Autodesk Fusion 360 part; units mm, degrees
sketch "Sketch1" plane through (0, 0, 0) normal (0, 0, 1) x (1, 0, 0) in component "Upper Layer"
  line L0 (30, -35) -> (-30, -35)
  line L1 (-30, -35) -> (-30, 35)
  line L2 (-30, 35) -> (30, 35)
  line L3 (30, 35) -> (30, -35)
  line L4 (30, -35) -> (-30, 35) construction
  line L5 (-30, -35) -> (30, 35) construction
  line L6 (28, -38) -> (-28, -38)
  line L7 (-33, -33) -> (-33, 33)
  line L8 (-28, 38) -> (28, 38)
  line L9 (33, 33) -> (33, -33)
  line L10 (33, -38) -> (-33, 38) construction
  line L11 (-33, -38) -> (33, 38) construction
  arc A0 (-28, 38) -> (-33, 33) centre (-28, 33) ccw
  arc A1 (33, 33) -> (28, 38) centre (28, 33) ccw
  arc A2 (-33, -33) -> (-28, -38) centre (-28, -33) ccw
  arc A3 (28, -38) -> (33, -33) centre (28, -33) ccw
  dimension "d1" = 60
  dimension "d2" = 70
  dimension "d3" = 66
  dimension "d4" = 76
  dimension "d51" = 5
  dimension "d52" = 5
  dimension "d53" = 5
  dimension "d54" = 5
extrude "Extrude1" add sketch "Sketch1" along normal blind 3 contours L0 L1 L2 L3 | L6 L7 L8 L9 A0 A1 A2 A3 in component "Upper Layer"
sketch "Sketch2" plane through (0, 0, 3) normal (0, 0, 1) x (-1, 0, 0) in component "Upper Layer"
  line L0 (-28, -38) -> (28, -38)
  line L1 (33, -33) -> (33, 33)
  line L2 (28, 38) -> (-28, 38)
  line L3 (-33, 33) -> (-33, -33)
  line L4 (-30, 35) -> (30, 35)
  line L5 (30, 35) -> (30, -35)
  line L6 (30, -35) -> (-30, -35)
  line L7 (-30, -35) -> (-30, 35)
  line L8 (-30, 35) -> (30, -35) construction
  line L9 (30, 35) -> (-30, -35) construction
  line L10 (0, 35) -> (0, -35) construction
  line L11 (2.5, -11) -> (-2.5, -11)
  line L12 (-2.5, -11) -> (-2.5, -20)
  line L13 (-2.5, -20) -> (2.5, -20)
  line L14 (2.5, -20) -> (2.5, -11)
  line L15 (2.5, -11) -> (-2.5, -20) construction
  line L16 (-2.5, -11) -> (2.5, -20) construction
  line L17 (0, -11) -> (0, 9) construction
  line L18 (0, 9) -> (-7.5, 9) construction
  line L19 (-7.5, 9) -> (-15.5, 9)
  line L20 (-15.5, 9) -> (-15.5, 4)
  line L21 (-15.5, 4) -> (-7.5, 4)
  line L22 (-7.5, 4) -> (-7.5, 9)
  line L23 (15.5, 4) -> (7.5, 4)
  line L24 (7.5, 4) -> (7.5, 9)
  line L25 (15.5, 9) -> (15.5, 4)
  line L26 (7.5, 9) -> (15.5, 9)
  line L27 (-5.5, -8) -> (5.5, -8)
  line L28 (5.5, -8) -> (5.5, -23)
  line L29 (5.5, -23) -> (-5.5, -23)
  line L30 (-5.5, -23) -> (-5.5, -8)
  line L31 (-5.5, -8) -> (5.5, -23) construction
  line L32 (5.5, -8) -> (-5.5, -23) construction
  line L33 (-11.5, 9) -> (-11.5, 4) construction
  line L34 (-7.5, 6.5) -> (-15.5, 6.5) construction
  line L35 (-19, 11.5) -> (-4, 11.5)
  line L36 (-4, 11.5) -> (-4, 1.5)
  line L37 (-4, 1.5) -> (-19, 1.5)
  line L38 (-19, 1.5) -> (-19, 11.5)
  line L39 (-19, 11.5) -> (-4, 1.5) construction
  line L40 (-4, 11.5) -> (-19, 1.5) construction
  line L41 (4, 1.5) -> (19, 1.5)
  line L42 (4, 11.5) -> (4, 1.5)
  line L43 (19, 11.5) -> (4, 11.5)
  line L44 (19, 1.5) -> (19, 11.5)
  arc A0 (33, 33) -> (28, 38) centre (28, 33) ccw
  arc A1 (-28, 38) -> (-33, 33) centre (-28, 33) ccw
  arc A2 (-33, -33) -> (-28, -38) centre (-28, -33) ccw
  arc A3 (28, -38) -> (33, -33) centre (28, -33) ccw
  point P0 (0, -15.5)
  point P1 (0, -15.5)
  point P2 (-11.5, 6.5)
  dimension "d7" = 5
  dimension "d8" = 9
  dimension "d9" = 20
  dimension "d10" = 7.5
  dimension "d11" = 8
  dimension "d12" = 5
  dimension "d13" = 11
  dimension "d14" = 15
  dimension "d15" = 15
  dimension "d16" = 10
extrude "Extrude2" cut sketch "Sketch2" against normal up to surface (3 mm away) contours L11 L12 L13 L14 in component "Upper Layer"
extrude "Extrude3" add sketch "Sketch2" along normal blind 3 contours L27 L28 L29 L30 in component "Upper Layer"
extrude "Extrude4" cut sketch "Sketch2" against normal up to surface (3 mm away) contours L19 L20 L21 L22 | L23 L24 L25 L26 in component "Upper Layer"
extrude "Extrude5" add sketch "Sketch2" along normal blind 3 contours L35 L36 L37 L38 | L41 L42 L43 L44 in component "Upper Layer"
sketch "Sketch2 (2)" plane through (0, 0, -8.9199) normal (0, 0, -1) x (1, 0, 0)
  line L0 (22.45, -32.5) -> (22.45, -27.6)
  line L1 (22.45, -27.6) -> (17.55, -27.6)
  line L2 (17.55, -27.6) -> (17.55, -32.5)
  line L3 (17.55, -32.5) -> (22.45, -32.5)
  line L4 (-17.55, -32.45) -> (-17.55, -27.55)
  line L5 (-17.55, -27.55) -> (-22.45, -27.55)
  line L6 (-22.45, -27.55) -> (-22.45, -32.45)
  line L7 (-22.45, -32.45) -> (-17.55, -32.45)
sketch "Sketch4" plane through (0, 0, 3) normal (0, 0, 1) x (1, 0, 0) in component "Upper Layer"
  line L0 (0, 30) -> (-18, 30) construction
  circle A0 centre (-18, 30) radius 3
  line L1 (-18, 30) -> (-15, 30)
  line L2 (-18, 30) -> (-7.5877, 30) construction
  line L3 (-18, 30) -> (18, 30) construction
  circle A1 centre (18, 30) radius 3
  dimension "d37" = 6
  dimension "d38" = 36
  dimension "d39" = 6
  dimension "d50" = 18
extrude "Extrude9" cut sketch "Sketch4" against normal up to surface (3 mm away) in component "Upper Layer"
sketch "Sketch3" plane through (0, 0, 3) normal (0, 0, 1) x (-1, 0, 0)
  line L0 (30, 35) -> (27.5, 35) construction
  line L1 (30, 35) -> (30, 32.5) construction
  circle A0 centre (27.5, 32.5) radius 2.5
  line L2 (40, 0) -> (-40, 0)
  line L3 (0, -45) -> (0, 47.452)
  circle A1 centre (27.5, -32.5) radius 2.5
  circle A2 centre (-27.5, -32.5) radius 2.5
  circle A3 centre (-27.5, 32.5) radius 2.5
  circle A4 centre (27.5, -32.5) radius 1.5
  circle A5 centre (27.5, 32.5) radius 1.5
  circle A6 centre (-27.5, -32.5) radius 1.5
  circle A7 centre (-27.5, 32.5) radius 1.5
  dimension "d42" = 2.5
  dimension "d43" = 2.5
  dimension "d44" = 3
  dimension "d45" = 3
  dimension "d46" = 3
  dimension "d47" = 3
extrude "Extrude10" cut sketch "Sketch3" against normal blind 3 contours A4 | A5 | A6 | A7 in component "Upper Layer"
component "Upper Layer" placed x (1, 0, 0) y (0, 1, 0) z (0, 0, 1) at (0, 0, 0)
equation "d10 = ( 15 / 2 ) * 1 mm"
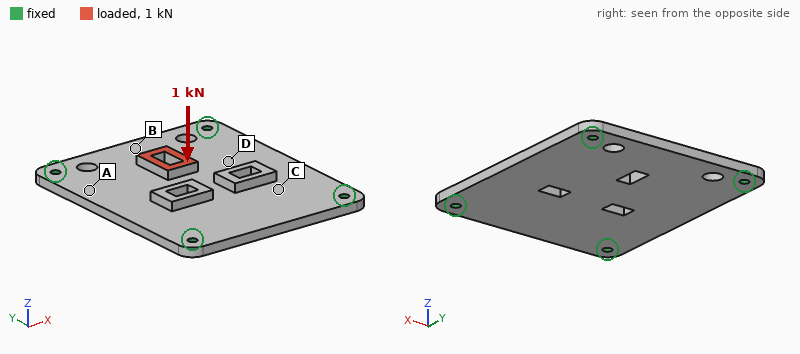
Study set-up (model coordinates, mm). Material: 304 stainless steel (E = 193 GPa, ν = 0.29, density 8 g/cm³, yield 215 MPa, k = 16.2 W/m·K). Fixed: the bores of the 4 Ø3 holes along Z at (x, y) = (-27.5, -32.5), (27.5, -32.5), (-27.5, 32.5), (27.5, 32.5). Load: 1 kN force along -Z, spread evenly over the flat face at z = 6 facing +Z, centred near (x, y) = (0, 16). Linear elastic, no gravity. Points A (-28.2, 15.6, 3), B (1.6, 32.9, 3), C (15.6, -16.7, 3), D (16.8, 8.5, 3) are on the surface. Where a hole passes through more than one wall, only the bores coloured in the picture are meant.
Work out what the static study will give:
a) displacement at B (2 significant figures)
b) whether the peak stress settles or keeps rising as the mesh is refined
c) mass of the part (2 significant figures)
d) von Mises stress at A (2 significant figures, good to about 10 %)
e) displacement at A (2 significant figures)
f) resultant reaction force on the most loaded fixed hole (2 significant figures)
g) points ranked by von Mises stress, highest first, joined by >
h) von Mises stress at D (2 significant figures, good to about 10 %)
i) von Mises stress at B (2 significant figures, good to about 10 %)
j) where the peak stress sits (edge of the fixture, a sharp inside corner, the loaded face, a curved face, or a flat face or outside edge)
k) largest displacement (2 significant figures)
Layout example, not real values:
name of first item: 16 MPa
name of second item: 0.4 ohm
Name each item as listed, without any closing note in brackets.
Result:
displacement at B: 49 µm
whether the peak stress settles or keeps rising as the mesh is refined: keeps rising
mass of the part: 120 g
von Mises stress at A: 25 MPa
displacement at A: 24 µm
resultant reaction force on the most loaded fixed hole: 390 N
points ranked by von Mises stress, highest first, joined by >: B > D > A > C
von Mises stress at D: 50 MPa
von Mises stress at B: 68 MPa
where the peak stress sits: edge of the fixture
largest displacement: 82 µm
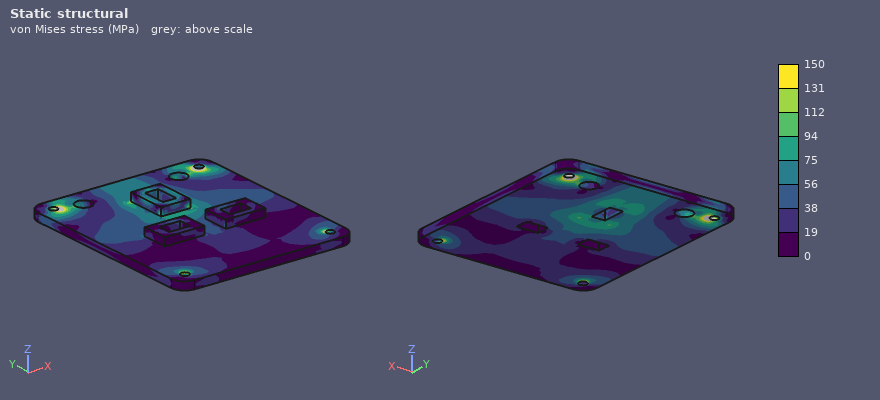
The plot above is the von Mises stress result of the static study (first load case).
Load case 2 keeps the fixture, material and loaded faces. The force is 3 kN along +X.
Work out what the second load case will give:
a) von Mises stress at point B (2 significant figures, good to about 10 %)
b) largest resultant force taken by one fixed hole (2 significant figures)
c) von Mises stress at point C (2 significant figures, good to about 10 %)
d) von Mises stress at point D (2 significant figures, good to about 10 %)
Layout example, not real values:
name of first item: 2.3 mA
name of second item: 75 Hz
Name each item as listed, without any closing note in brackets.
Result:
von Mises stress at point B: 47 MPa
largest resultant force taken by one fixed hole: 1.1 kN
von Mises stress at point C: 23 MPa
von Mises stress at point D: 36 MPa
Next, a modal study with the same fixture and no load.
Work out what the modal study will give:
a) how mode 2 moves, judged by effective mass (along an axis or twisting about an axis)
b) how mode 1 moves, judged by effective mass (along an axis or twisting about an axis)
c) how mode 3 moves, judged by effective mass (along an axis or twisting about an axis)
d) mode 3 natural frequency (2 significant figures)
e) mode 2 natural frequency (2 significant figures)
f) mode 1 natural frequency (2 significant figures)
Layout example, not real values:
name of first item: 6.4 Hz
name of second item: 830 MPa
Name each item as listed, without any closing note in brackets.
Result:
how mode 2 moves, judged by effective mass: twisting about Y
how mode 1 moves, judged by effective mass: along Z
how mode 3 moves, judged by effective mass: twisting about X
mode 3 natural frequency: 5000 Hz
mode 2 natural frequency: 4100 Hz
mode 1 natural frequency: 2500 Hz
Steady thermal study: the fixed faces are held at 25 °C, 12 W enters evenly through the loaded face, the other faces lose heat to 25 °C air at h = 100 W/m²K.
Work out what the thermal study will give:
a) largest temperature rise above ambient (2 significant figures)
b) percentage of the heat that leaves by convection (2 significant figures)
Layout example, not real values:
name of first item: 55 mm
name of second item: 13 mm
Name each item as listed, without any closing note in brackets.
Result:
largest temperature rise above ambient: 65 K
percentage of the heat that leaves by convection: 89 %
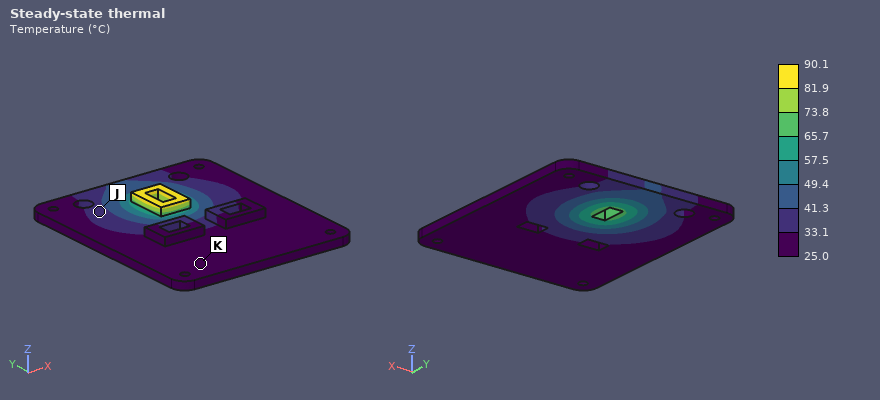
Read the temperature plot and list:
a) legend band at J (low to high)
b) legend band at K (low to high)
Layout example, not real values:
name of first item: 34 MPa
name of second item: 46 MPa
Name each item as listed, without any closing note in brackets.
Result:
legend band at J: 33.1 to 41.3 °C
legend band at K: 25.0 to 33.1 °C
